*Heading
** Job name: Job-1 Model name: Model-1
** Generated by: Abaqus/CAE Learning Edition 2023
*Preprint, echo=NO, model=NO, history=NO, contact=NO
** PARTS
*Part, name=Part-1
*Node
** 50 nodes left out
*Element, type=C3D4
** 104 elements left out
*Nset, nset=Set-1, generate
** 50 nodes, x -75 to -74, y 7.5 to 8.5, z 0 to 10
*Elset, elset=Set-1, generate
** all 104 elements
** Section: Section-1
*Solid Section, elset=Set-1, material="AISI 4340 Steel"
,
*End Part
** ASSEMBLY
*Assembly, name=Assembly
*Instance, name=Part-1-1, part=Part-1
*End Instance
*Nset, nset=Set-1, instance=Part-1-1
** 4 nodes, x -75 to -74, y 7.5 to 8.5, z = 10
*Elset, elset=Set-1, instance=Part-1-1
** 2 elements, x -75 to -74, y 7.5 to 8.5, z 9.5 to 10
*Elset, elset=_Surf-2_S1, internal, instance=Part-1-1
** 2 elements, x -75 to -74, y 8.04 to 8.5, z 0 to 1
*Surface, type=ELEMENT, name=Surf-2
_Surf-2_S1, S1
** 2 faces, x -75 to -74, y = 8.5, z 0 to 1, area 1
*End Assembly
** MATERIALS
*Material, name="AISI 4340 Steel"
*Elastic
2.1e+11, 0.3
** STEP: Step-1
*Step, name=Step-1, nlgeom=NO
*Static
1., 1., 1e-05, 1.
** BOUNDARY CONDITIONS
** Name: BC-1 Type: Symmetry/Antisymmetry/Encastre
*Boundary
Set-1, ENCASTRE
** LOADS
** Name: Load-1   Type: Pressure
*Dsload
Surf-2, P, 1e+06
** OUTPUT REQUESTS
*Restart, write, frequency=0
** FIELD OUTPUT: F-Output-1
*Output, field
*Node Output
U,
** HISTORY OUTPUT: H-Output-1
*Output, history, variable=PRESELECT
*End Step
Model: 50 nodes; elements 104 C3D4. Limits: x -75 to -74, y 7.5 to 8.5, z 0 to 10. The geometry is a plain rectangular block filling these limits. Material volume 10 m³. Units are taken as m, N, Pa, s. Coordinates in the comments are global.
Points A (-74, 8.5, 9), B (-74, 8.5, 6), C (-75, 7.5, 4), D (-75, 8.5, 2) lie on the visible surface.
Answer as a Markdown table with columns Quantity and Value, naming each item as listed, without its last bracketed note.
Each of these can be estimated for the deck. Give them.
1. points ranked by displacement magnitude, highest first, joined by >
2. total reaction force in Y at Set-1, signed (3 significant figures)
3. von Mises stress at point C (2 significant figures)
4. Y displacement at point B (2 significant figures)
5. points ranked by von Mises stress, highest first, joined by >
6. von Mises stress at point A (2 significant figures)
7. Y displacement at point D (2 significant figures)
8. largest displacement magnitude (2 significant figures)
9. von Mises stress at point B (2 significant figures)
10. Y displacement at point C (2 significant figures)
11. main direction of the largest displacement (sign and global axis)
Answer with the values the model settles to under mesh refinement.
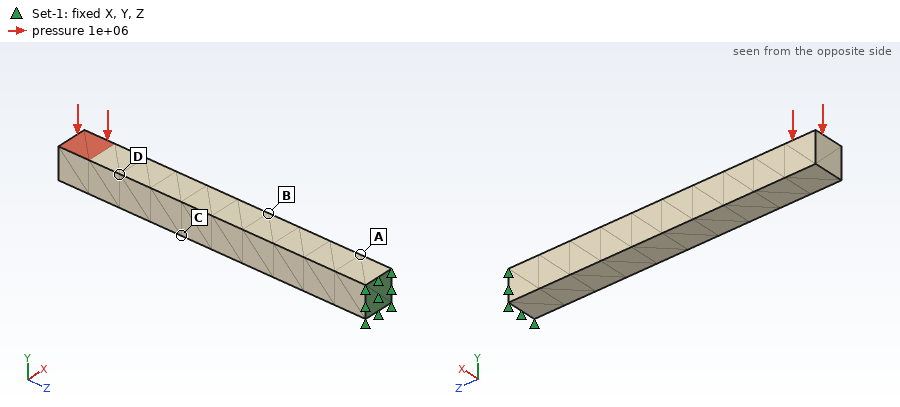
| Quantity | Value |
|---|---|
| points ranked by displacement magnitude, highest first, joined by > | D > C > B > A |
| total reaction force in Y at Set-1, signed | 1.00e+06 N |
| von Mises stress at point C | 2.1e+07 Pa |
| Y displacement at point B | -0.0037 m |
| points ranked by von Mises stress, highest first, joined by > | A > B > C > D |
| von Mises stress at point A | 5.1e+07 Pa |
| Y displacement at point D | -0.012 m |
| largest displacement magnitude | 0.018 m |
| von Mises stress at point B | 3.2e+07 Pa |
| Y displacement at point C | -0.0077 m |
| main direction of the largest displacement | -Y |
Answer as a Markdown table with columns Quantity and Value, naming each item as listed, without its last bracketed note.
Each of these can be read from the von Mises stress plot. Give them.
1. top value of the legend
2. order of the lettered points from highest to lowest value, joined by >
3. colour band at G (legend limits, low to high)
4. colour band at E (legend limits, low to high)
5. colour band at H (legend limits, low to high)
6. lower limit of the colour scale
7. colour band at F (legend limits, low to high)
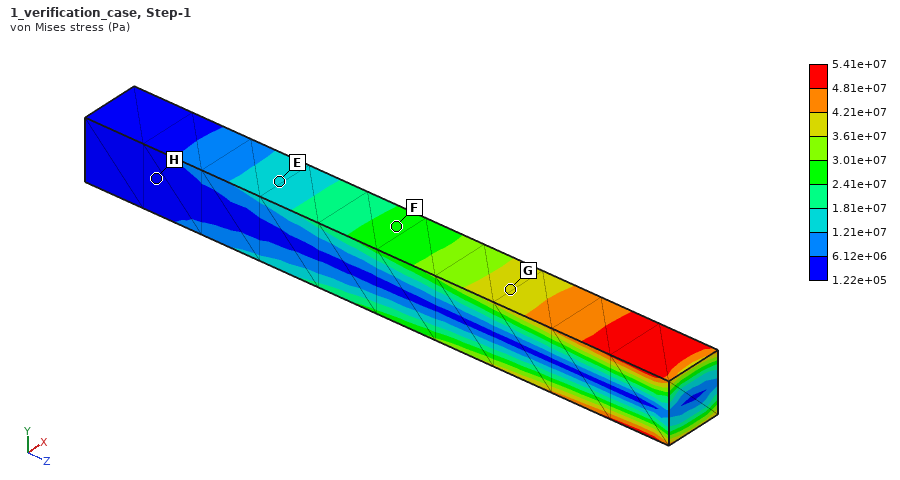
| Quantity | Value |
|---|---|
| top value of the legend | 5.41e+07 Pa |
| order of the lettered points from highest to lowest value, joined by > | G > F > E > H |
| colour band at G | 3.61e+07 to 4.21e+07 Pa |
| colour band at E | 1.21e+07 to 1.81e+07 Pa |
| colour band at H | 1.22e+05 to 6.12e+06 Pa |
| lower limit of the colour scale | 1.22e+05 Pa |
| colour band at F | 2.41e+07 to 3.01e+07 Pa |
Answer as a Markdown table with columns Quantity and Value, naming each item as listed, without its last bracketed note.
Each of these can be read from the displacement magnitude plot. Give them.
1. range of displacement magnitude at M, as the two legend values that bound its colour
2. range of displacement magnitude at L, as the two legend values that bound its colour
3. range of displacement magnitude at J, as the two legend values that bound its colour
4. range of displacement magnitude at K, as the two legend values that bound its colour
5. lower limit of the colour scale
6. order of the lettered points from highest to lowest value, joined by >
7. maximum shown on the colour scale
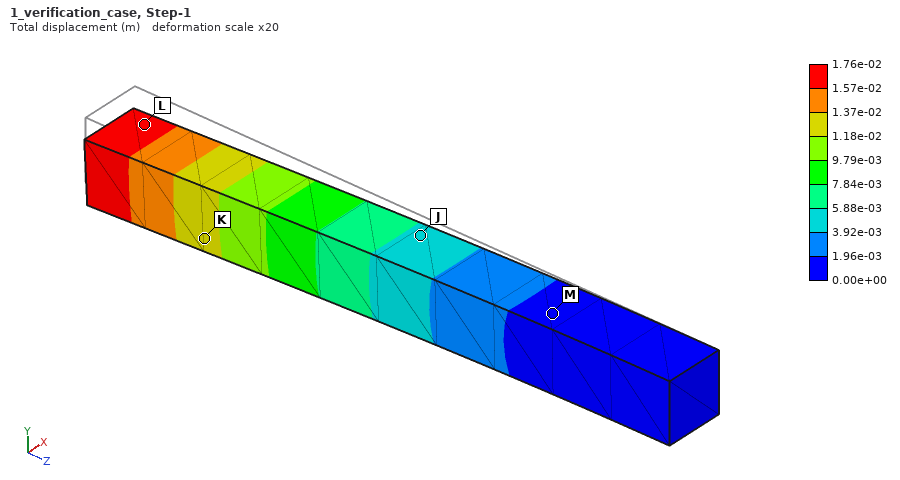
| Quantity | Value |
|---|---|
| range of displacement magnitude at M, as the two legend values that bound its colour | 0.00e+00 to 1.96e-03 m |
| range of displacement magnitude at L, as the two legend values that bound its colour | 1.57e-02 to 1.76e-02 m |
| range of displacement magnitude at J, as the two legend values that bound its colour | 3.92e-03 to 5.88e-03 m |
| range of displacement magnitude at K, as the two legend values that bound its colour | 1.18e-02 to 1.37e-02 m |
| lower limit of the colour scale | 0.00e+00 m |
| order of the lettered points from highest to lowest value, joined by > | L > K > J > M |
| maximum shown on the colour scale | 1.76e-02 m |
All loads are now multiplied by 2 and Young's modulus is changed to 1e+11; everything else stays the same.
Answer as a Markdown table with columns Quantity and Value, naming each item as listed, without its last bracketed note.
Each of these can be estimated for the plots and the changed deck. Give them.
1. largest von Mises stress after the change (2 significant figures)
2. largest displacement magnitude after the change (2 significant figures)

| Quantity | Value |
|---|---|
| largest von Mises stress after the change | 1.1e+08 Pa |
| largest displacement magnitude after the change | 0.074 m |
